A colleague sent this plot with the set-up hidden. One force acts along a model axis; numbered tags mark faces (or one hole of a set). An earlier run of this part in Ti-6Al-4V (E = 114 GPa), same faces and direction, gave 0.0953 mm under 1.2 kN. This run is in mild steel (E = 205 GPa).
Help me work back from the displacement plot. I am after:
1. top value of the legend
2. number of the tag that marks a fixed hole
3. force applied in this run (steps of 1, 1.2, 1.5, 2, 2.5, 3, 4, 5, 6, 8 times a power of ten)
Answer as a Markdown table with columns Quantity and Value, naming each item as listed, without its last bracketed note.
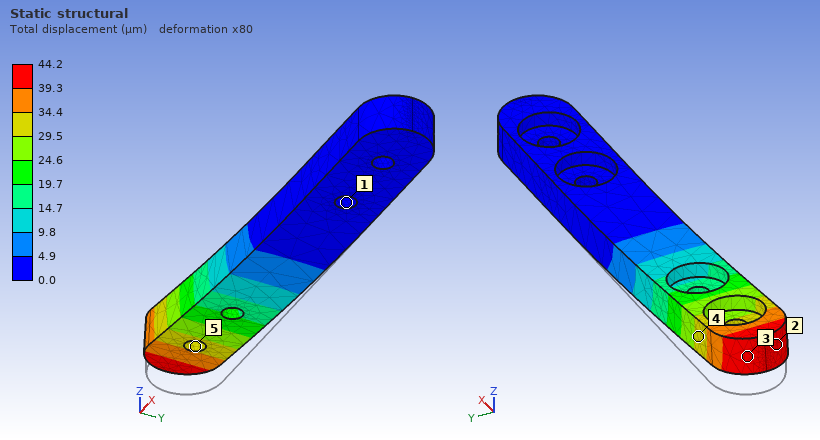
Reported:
| Quantity | Value |
|---|---|
| top value of the legend | 44.2 µm |
| number of the tag that marks a fixed hole | 1 |
| force applied in this run | 1 kN |
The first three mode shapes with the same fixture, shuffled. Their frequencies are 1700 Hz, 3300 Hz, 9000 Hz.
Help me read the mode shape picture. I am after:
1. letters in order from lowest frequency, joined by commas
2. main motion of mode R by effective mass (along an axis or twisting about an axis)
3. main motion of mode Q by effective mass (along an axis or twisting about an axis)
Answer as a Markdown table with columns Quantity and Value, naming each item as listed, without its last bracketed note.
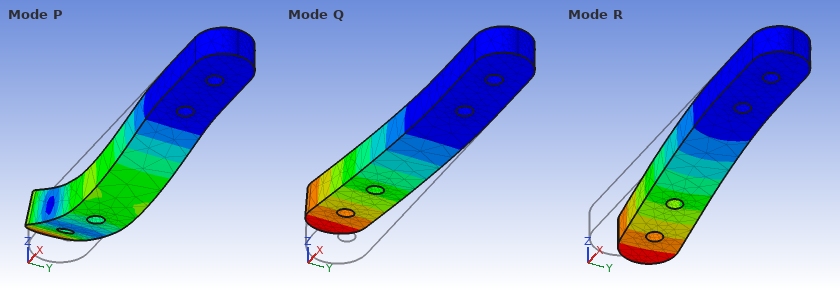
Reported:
| Quantity | Value |
|---|---|
| letters in order from lowest frequency, joined by commas | Q, R, P |
| main motion of mode R by effective mass | along Y |
| main motion of mode Q by effective mass | along Z |
